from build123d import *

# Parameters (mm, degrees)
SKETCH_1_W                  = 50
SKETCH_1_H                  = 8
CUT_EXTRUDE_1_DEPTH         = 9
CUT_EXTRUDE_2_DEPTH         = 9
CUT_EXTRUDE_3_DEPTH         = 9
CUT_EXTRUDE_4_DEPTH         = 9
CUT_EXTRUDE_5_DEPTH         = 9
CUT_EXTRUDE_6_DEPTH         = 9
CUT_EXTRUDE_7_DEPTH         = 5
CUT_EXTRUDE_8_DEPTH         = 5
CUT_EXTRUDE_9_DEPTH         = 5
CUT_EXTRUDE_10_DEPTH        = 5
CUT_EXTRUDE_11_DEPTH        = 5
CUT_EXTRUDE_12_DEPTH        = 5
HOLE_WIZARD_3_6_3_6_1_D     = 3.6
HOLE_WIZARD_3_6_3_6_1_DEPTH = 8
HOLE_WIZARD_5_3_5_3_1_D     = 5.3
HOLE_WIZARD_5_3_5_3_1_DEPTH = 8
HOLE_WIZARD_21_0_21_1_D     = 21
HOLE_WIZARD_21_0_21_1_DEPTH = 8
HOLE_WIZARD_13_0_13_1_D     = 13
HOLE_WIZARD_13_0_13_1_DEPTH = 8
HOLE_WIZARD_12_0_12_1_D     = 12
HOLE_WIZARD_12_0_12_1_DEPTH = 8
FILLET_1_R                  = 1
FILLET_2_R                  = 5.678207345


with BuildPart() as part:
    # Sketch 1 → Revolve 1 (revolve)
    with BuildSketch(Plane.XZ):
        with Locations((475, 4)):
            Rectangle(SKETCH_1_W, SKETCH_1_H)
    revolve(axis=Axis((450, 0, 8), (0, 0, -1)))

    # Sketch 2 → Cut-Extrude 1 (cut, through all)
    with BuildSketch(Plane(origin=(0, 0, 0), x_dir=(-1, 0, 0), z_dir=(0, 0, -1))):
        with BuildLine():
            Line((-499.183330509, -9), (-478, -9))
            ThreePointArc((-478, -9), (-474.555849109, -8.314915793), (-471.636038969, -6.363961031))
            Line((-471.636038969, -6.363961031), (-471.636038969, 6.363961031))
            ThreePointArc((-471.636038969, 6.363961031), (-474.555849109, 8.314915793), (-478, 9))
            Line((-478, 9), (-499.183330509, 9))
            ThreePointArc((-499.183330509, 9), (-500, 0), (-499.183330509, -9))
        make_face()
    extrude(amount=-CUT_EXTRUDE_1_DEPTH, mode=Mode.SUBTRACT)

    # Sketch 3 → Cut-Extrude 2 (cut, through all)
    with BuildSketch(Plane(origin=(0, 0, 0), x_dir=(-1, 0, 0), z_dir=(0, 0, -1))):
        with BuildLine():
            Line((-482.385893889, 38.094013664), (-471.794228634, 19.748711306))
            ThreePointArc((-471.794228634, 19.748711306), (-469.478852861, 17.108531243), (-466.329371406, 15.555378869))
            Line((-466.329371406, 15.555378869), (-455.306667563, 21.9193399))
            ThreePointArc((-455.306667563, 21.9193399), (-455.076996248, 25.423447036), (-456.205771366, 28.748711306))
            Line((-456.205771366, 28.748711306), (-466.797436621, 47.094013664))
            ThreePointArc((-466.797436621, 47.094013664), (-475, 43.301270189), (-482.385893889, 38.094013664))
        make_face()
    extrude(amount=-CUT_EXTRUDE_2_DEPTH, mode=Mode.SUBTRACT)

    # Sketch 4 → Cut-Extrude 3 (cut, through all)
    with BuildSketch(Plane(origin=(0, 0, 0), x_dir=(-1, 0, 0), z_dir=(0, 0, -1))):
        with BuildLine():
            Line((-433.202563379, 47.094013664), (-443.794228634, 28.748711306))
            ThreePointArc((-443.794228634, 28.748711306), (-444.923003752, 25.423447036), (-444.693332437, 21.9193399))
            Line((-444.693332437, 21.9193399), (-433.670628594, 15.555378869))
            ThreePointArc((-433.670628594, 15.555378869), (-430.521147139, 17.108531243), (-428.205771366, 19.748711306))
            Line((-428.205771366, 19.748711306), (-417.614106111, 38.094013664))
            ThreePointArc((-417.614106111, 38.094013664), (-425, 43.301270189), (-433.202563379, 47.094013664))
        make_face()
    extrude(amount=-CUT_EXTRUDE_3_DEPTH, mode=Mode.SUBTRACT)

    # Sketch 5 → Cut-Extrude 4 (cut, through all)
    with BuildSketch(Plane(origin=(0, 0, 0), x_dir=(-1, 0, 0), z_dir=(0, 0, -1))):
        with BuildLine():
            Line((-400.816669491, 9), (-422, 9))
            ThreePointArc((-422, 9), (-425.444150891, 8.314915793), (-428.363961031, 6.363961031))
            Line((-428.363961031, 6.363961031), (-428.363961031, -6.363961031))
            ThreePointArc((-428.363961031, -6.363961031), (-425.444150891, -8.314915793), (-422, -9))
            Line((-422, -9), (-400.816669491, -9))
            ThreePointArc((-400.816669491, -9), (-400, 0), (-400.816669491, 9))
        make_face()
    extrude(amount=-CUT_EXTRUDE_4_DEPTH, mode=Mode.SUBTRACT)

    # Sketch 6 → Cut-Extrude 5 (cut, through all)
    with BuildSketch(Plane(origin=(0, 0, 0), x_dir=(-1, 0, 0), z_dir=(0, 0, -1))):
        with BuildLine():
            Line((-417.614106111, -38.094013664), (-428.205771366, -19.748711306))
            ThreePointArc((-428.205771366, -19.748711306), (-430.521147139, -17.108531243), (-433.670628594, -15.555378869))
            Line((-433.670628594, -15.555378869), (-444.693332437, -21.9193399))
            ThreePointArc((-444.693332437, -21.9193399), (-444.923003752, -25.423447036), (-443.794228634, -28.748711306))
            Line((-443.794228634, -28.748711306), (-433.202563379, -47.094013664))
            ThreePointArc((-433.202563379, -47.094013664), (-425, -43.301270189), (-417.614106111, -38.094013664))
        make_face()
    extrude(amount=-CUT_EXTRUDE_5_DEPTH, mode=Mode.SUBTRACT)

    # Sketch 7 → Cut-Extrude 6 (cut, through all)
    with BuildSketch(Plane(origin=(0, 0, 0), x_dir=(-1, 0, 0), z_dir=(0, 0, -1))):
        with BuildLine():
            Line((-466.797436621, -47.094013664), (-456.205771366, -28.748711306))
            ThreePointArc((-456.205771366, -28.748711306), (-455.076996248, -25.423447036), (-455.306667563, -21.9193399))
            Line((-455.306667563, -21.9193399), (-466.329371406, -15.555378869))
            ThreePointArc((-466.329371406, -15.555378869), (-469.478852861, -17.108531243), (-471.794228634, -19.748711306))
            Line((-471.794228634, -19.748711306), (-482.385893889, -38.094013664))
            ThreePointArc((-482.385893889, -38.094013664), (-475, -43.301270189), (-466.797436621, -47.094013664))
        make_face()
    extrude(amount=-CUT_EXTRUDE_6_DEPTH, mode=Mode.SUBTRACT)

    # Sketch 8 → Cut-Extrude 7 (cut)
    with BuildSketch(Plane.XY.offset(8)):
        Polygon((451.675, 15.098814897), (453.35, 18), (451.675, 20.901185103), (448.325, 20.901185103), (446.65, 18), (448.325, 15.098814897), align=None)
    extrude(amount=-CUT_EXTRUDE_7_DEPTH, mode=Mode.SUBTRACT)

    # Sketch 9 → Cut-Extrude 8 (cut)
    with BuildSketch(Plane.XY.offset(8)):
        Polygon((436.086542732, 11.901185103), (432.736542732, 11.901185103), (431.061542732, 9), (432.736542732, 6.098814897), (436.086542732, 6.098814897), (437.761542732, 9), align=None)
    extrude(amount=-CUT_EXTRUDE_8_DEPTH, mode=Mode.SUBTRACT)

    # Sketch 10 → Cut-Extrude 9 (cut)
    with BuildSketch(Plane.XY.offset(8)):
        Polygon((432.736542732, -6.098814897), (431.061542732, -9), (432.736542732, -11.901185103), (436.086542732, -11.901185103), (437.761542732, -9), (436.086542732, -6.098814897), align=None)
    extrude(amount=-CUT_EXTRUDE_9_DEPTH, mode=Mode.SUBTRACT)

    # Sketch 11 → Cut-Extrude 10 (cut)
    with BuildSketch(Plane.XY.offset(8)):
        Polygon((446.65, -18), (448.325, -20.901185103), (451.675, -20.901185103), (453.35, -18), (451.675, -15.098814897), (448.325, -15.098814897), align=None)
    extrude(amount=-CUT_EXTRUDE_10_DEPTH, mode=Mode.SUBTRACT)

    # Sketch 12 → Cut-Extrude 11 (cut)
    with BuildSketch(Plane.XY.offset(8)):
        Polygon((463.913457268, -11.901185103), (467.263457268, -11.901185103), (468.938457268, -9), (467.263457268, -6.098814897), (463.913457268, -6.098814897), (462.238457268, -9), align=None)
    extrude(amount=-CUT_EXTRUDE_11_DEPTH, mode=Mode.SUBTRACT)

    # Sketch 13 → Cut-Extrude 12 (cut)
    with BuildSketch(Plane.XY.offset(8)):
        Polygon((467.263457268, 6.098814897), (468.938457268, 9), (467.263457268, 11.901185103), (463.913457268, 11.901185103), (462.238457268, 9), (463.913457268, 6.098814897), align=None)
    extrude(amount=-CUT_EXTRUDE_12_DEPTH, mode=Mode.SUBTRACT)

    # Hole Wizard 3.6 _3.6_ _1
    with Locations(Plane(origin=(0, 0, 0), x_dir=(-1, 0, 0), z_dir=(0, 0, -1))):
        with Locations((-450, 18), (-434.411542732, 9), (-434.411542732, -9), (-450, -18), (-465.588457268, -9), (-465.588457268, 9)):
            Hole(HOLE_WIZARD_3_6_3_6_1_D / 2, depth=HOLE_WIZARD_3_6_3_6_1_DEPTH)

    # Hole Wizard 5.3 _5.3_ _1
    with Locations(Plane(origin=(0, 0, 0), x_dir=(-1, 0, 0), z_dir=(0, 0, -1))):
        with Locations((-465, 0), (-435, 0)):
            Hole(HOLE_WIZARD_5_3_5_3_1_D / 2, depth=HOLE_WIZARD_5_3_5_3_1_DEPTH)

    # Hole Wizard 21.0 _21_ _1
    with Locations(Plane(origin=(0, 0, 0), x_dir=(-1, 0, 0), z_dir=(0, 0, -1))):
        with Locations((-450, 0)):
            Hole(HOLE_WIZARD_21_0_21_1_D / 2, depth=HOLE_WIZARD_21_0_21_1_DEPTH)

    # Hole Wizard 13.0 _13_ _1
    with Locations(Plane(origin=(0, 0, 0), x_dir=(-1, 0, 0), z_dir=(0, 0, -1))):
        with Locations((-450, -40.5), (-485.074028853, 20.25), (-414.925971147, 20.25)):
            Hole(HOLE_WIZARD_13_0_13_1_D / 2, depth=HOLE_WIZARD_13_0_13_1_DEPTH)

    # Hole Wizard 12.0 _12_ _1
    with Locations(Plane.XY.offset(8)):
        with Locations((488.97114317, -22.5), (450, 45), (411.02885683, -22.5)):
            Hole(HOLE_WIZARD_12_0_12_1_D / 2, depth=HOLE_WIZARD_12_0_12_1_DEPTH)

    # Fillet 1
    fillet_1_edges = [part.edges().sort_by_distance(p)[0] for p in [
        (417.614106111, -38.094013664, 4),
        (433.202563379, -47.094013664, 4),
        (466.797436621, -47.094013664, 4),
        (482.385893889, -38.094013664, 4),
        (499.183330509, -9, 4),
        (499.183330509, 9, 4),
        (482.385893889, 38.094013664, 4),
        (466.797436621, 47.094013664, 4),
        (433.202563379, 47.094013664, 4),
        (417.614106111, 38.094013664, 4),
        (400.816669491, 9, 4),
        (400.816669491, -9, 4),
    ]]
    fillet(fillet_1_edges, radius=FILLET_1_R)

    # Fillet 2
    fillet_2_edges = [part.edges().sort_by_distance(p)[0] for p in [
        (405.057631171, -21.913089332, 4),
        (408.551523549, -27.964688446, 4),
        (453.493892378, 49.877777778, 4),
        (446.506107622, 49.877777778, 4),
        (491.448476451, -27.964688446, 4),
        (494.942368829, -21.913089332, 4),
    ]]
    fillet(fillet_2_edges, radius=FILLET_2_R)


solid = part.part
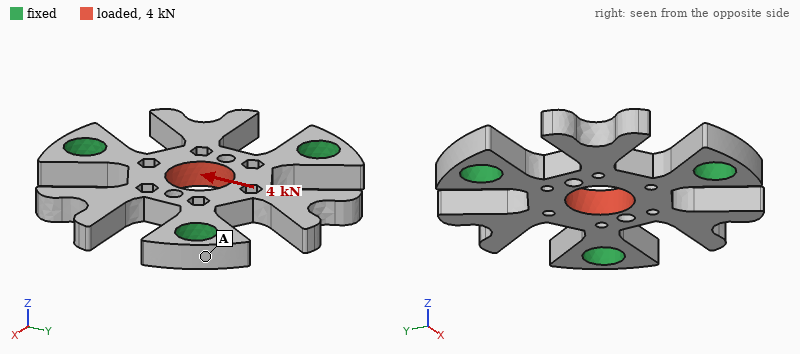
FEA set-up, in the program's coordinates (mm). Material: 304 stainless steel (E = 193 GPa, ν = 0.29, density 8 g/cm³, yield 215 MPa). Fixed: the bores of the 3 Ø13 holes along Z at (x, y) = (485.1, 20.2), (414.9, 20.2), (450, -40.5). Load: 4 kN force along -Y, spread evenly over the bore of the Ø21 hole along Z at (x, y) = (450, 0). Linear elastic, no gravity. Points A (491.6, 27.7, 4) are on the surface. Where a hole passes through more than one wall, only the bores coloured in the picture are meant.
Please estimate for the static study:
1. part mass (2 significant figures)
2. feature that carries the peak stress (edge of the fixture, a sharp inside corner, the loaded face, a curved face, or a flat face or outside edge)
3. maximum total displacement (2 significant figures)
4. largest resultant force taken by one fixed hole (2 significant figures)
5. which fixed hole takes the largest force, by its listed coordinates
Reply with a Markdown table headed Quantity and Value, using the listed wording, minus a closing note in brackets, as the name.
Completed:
| Quantity | Value |
|---|---|
| part mass | 230 g |
| feature that carries the peak stress | a curved face |
| maximum total displacement | 8.0 µm |
| largest resultant force taken by one fixed hole | 1.9 kN |
| which fixed hole takes the largest force, by its listed coordinates | (450, -40.5) |
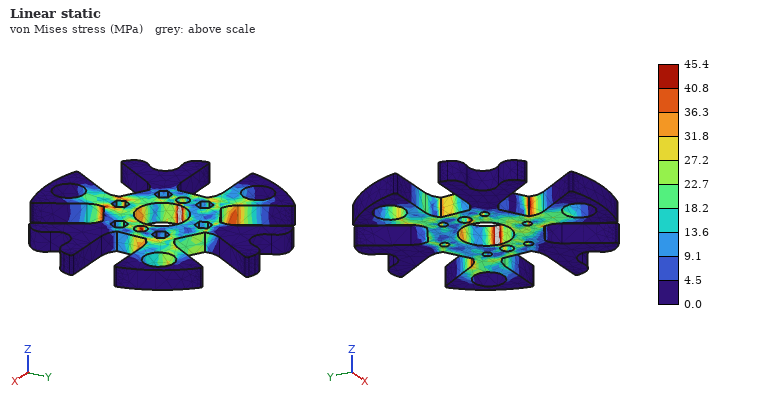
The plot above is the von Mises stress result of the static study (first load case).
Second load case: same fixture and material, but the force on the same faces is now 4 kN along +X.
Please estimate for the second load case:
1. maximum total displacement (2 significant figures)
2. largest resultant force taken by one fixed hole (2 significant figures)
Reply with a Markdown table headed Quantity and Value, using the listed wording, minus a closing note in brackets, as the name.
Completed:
| Quantity | Value |
|---|---|
| maximum total displacement | 8.3 µm |
| largest resultant force taken by one fixed hole | 1.5 kN |
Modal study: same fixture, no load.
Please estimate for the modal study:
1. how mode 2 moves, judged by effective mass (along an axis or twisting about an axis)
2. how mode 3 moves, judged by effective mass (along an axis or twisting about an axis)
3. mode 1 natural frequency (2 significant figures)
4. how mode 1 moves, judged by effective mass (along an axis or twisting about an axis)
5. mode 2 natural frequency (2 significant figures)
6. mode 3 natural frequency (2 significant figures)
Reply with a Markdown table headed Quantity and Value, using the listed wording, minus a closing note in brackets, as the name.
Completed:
| Quantity | Value |
|---|---|
| how mode 2 moves, judged by effective mass | twisting about X |
| how mode 3 moves, judged by effective mass | along Z |
| mode 1 natural frequency | 2300 Hz |
| how mode 1 moves, judged by effective mass | twisting about Y |
| mode 2 natural frequency | 2400 Hz |
| mode 3 natural frequency | 2800 Hz |
